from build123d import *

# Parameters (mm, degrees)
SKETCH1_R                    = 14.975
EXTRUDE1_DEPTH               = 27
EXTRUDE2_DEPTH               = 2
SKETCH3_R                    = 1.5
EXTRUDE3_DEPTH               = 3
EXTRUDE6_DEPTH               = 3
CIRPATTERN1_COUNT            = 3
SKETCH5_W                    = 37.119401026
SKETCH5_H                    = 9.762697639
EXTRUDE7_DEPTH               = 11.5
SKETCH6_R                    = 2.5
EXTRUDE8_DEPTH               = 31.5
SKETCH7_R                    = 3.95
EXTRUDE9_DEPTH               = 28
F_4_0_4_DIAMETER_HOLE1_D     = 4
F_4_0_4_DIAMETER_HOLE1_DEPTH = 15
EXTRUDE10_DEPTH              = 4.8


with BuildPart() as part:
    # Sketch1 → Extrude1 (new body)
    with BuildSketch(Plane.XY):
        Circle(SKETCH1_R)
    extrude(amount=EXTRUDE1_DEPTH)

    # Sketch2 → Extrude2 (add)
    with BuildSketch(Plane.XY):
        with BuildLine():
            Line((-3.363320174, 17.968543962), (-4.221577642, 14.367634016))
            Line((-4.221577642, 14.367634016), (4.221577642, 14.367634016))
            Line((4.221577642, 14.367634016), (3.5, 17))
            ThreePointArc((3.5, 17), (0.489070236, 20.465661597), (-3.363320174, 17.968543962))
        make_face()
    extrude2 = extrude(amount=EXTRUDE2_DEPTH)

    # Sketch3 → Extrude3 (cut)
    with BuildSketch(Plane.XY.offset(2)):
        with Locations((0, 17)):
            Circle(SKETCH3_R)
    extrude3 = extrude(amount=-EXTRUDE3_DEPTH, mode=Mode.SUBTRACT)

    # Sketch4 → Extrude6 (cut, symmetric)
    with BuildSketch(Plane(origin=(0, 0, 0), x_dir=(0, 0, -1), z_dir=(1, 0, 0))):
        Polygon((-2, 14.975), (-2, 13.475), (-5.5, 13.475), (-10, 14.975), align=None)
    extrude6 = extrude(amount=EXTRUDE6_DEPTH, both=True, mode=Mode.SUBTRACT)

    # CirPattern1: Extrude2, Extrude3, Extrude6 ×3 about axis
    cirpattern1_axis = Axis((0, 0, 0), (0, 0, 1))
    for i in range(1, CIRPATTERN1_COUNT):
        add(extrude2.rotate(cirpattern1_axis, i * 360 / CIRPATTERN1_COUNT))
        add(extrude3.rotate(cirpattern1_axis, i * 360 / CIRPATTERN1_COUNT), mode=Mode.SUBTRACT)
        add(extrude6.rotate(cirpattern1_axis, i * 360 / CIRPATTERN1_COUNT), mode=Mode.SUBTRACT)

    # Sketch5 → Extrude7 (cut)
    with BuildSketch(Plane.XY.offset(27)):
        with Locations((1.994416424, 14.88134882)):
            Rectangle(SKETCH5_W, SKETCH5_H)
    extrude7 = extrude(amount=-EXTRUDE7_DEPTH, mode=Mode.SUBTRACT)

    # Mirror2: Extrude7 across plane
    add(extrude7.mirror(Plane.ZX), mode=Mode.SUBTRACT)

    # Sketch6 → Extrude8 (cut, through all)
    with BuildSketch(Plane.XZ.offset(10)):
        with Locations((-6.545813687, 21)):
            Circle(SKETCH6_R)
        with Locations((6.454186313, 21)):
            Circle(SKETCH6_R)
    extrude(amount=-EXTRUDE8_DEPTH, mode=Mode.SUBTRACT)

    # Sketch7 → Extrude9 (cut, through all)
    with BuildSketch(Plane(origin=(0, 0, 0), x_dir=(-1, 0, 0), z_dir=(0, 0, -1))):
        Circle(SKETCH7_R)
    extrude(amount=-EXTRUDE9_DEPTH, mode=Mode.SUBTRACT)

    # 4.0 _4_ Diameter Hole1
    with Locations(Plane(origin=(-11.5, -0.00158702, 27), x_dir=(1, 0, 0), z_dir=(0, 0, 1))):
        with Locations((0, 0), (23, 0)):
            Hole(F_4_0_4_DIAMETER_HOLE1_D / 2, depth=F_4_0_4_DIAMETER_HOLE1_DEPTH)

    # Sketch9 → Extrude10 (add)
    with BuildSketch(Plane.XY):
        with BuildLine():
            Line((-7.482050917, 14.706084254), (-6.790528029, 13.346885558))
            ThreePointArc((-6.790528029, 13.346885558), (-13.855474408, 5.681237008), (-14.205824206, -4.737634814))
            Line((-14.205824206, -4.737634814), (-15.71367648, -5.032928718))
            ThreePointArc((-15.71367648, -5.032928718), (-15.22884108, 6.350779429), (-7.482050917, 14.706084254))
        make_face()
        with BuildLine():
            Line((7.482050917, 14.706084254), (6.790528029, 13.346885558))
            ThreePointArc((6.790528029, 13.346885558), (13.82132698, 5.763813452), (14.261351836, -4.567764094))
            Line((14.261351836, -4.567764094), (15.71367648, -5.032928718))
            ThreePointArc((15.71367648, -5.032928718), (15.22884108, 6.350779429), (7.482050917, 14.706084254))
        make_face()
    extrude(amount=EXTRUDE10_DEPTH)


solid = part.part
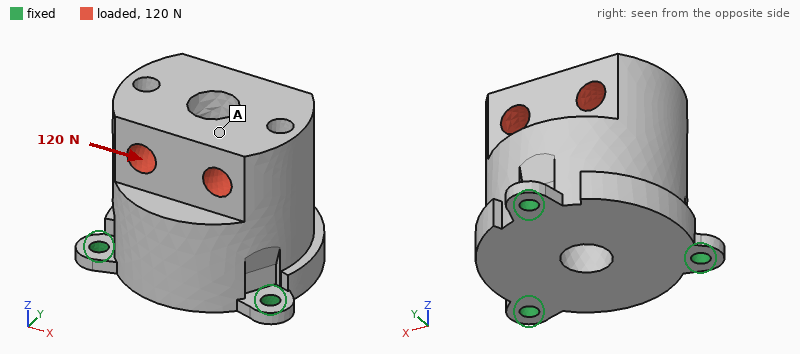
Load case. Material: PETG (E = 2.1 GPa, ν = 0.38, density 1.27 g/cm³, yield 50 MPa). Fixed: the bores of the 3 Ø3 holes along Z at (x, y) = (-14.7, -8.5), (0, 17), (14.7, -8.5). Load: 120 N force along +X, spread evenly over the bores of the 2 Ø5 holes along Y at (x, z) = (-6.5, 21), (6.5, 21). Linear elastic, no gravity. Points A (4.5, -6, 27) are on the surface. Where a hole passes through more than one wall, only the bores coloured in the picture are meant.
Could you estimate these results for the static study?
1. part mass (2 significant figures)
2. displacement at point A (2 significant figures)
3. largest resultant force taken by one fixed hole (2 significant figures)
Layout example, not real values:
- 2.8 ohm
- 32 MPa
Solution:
- 19 g
- 0.12 mm
- 110 N
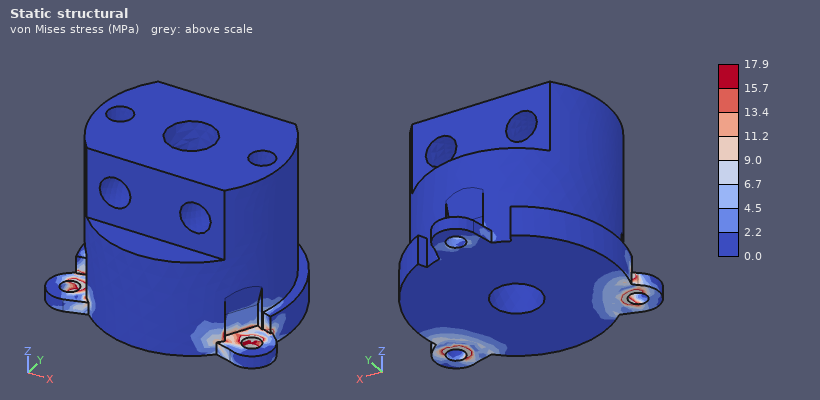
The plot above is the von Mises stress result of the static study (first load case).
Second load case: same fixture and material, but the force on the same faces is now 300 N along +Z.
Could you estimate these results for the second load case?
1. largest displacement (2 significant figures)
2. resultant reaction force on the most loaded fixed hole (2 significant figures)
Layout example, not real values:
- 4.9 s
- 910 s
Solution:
- 69 µm
- 110 N
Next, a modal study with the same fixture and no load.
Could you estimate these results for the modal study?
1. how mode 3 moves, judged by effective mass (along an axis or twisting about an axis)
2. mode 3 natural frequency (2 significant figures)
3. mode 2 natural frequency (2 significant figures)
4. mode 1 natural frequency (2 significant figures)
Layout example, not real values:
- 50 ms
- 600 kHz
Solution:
- along Z
- 2600 Hz
- 1700 Hz
- 1700 Hz
